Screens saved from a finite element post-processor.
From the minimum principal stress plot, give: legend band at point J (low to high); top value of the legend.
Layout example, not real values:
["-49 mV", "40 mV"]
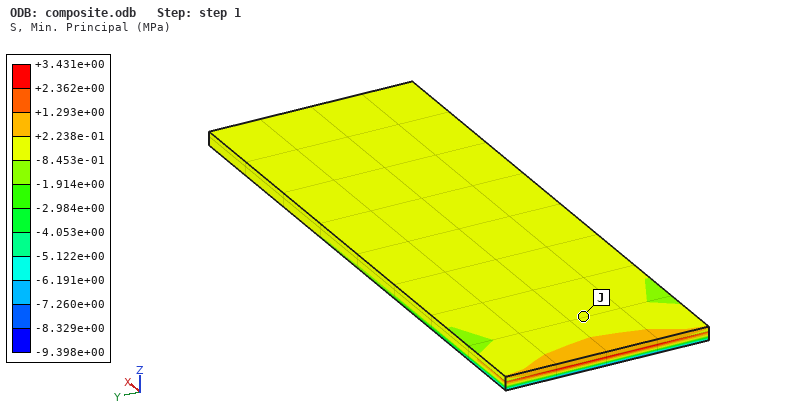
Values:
["-8.453e-01 to +2.238e-01 MPa", "+3.431e+00 MPa"]
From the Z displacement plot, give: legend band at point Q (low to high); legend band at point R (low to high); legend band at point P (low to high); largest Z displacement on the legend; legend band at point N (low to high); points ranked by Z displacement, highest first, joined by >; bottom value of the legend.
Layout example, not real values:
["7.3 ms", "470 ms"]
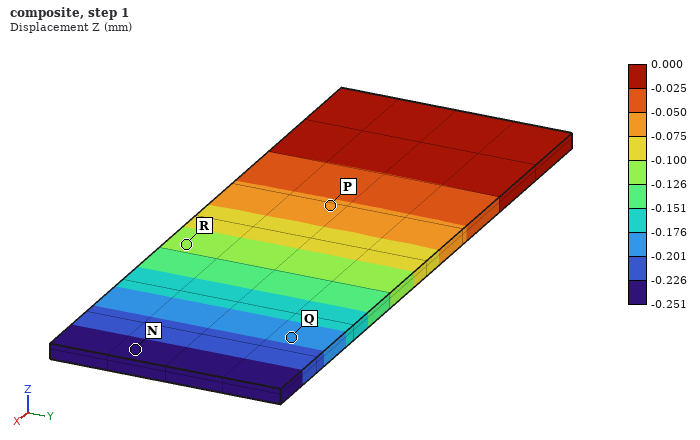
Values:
["-0.201 to -0.176 mm", "-0.126 to -0.100 mm", "-0.075 to -0.050 mm", "0.000 mm", "-0.251 to -0.226 mm", "P > R > Q > N", "-0.251 mm"]
